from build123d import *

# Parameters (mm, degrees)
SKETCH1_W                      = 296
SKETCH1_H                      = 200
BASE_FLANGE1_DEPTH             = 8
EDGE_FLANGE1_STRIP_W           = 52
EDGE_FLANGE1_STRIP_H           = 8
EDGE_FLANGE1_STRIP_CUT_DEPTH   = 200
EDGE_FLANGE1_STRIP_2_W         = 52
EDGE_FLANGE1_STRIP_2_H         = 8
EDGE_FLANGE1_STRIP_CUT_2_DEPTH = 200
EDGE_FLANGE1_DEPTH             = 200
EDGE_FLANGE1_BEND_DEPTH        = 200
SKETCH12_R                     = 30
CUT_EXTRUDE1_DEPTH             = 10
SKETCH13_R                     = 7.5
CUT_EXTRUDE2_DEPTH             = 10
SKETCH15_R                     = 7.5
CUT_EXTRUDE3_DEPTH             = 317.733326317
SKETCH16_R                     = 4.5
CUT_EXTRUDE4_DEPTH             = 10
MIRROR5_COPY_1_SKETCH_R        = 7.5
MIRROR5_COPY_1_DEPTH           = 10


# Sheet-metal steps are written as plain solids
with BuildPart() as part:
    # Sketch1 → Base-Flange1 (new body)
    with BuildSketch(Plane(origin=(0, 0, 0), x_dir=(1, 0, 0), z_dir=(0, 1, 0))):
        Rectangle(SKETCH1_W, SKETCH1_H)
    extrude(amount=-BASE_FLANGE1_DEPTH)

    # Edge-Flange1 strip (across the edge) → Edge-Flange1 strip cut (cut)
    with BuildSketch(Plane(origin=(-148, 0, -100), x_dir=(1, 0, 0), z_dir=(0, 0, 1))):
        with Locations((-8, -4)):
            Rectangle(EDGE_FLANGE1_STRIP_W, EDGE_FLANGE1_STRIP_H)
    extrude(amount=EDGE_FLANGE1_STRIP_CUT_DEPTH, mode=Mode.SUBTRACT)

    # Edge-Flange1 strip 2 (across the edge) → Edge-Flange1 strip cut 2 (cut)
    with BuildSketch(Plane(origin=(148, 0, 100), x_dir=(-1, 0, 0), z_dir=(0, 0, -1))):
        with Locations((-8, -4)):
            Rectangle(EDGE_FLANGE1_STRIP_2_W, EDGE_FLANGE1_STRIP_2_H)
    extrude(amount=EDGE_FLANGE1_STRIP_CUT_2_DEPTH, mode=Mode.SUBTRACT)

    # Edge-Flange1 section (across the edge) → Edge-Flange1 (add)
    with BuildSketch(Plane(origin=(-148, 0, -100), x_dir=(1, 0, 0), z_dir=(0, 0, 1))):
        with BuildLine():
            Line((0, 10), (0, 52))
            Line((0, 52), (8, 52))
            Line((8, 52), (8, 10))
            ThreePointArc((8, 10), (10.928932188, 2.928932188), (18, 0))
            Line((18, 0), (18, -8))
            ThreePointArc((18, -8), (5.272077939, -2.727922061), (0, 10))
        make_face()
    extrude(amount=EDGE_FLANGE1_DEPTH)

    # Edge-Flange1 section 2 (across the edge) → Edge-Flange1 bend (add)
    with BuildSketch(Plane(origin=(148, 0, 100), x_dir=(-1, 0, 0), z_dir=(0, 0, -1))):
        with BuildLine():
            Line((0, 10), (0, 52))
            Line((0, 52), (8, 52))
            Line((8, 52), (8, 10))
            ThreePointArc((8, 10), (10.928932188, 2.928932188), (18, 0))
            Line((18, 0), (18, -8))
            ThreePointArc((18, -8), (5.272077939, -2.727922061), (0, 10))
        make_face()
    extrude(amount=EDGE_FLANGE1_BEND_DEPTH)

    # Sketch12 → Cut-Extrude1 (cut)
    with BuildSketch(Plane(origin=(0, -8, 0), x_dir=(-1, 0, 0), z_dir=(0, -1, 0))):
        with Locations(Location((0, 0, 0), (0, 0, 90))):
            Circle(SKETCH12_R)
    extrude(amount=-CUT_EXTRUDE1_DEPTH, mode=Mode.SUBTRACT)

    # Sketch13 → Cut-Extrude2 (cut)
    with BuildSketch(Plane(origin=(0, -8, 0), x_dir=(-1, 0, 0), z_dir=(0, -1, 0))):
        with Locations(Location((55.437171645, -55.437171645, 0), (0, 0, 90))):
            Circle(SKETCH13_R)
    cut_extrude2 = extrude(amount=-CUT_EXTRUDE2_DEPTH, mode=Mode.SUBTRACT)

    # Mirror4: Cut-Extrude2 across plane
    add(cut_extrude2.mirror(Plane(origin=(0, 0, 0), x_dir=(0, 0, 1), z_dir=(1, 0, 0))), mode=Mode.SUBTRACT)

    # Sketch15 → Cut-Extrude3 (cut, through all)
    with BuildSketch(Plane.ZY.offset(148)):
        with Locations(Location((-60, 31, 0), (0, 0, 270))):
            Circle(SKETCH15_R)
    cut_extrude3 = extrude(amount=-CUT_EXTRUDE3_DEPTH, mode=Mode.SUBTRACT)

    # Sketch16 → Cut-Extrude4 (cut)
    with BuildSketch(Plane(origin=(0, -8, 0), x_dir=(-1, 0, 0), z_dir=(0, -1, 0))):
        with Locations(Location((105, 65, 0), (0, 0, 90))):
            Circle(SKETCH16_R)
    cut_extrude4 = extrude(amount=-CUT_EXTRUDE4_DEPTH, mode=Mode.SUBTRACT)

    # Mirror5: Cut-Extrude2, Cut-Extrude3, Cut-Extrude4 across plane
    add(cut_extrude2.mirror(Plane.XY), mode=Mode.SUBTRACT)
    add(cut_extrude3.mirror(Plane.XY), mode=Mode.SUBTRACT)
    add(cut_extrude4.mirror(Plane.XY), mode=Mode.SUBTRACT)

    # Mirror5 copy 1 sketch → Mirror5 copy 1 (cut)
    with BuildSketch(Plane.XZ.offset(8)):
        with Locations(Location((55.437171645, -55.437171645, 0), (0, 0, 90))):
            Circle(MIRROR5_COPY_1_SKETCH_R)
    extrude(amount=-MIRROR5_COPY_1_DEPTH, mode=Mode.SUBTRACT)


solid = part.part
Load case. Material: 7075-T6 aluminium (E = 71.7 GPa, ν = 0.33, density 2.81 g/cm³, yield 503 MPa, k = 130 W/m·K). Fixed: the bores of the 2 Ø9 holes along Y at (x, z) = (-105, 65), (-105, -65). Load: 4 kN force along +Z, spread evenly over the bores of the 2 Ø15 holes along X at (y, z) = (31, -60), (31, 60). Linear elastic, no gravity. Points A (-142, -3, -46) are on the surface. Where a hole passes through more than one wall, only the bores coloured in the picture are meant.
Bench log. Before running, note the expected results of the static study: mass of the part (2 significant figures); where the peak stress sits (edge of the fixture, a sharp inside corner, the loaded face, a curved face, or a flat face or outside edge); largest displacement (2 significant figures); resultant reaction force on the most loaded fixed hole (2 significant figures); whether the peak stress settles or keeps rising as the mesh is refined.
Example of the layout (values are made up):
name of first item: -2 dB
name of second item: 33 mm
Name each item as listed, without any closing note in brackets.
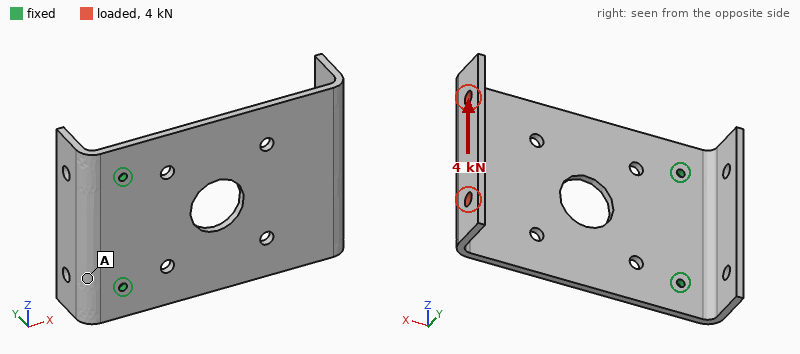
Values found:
mass of the part: 1.6 kg
where the peak stress sits: edge of the fixture
largest displacement: 3.7 mm
resultant reaction force on the most loaded fixed hole: 7.8 kN
whether the peak stress settles or keeps rising as the mesh is refined: keeps rising
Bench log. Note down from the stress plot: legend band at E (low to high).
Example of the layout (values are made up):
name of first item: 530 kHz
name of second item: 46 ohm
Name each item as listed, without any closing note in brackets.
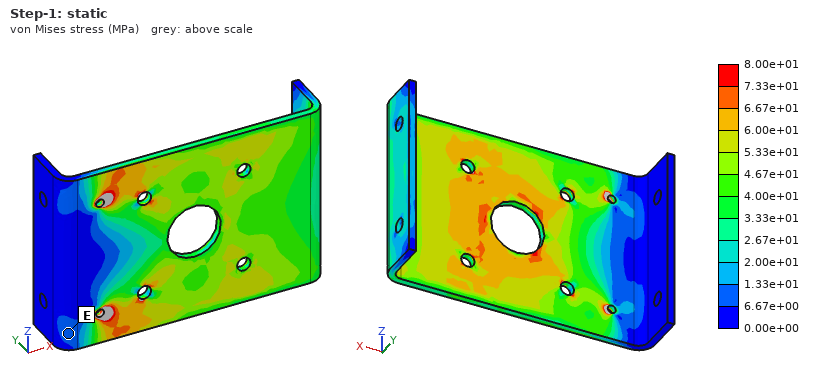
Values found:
legend band at E: 6.67e+00 to 1.33e+01 MPa
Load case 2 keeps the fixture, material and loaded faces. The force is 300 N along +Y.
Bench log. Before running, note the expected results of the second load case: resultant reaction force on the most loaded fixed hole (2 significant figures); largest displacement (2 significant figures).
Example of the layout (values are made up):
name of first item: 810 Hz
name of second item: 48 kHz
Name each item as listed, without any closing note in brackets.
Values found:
resultant reaction force on the most loaded fixed hole: 150 N
largest displacement: 3.3 mm
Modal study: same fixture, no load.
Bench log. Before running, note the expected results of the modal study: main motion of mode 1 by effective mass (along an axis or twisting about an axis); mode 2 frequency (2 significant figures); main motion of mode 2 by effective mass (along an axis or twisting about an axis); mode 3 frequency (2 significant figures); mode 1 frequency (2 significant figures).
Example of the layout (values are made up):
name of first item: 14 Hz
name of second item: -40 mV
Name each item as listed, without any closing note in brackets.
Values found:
main motion of mode 1 by effective mass: along Y
mode 2 frequency: 220 Hz
main motion of mode 2 by effective mass: twisting about X
mode 3 frequency: 460 Hz
mode 1 frequency: 71 Hz
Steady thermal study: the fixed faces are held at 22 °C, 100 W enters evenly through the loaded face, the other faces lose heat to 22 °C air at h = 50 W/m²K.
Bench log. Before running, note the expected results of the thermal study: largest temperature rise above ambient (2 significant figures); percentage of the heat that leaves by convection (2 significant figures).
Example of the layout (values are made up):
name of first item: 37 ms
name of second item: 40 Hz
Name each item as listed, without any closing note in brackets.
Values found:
largest temperature rise above ambient: 50 K
percentage of the heat that leaves by convection: 94 %
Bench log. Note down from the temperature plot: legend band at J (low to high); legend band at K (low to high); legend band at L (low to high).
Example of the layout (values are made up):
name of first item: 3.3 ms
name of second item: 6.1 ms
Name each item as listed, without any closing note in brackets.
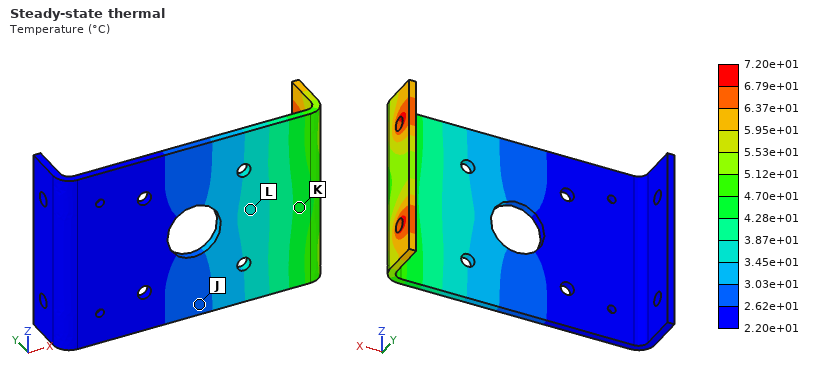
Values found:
legend band at J: 2.62e+01 to 3.03e+01 °C
legend band at K: 4.28e+01 to 4.70e+01 °C
legend band at L: 3.45e+01 to 3.87e+01 °C
